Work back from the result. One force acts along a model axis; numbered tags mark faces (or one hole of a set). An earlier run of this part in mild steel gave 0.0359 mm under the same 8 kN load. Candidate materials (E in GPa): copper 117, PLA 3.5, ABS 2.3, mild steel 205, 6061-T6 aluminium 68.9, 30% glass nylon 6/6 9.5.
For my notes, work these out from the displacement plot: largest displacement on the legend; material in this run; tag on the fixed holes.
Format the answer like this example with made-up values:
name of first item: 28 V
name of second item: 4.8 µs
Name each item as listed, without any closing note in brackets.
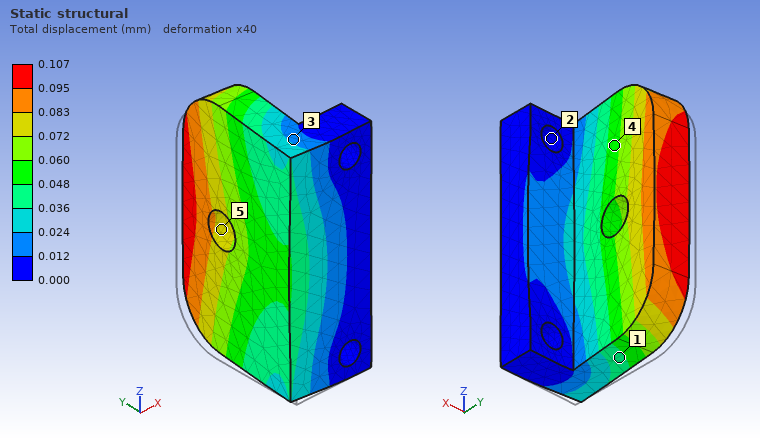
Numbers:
largest displacement on the legend: 0.107 mm
material in this run: 6061-T6 aluminium
tag on the fixed holes: 2
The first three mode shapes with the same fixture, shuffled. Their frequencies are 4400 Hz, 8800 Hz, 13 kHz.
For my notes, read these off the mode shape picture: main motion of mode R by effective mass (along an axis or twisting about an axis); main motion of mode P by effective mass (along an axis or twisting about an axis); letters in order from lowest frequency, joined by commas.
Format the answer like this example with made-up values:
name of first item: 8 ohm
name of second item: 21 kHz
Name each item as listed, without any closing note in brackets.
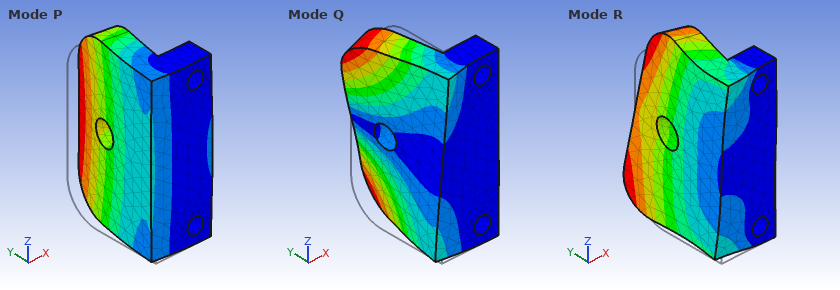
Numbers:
main motion of mode R by effective mass: along Z
main motion of mode P by effective mass: along X
letters in order from lowest frequency, joined by commas: P, Q, R
